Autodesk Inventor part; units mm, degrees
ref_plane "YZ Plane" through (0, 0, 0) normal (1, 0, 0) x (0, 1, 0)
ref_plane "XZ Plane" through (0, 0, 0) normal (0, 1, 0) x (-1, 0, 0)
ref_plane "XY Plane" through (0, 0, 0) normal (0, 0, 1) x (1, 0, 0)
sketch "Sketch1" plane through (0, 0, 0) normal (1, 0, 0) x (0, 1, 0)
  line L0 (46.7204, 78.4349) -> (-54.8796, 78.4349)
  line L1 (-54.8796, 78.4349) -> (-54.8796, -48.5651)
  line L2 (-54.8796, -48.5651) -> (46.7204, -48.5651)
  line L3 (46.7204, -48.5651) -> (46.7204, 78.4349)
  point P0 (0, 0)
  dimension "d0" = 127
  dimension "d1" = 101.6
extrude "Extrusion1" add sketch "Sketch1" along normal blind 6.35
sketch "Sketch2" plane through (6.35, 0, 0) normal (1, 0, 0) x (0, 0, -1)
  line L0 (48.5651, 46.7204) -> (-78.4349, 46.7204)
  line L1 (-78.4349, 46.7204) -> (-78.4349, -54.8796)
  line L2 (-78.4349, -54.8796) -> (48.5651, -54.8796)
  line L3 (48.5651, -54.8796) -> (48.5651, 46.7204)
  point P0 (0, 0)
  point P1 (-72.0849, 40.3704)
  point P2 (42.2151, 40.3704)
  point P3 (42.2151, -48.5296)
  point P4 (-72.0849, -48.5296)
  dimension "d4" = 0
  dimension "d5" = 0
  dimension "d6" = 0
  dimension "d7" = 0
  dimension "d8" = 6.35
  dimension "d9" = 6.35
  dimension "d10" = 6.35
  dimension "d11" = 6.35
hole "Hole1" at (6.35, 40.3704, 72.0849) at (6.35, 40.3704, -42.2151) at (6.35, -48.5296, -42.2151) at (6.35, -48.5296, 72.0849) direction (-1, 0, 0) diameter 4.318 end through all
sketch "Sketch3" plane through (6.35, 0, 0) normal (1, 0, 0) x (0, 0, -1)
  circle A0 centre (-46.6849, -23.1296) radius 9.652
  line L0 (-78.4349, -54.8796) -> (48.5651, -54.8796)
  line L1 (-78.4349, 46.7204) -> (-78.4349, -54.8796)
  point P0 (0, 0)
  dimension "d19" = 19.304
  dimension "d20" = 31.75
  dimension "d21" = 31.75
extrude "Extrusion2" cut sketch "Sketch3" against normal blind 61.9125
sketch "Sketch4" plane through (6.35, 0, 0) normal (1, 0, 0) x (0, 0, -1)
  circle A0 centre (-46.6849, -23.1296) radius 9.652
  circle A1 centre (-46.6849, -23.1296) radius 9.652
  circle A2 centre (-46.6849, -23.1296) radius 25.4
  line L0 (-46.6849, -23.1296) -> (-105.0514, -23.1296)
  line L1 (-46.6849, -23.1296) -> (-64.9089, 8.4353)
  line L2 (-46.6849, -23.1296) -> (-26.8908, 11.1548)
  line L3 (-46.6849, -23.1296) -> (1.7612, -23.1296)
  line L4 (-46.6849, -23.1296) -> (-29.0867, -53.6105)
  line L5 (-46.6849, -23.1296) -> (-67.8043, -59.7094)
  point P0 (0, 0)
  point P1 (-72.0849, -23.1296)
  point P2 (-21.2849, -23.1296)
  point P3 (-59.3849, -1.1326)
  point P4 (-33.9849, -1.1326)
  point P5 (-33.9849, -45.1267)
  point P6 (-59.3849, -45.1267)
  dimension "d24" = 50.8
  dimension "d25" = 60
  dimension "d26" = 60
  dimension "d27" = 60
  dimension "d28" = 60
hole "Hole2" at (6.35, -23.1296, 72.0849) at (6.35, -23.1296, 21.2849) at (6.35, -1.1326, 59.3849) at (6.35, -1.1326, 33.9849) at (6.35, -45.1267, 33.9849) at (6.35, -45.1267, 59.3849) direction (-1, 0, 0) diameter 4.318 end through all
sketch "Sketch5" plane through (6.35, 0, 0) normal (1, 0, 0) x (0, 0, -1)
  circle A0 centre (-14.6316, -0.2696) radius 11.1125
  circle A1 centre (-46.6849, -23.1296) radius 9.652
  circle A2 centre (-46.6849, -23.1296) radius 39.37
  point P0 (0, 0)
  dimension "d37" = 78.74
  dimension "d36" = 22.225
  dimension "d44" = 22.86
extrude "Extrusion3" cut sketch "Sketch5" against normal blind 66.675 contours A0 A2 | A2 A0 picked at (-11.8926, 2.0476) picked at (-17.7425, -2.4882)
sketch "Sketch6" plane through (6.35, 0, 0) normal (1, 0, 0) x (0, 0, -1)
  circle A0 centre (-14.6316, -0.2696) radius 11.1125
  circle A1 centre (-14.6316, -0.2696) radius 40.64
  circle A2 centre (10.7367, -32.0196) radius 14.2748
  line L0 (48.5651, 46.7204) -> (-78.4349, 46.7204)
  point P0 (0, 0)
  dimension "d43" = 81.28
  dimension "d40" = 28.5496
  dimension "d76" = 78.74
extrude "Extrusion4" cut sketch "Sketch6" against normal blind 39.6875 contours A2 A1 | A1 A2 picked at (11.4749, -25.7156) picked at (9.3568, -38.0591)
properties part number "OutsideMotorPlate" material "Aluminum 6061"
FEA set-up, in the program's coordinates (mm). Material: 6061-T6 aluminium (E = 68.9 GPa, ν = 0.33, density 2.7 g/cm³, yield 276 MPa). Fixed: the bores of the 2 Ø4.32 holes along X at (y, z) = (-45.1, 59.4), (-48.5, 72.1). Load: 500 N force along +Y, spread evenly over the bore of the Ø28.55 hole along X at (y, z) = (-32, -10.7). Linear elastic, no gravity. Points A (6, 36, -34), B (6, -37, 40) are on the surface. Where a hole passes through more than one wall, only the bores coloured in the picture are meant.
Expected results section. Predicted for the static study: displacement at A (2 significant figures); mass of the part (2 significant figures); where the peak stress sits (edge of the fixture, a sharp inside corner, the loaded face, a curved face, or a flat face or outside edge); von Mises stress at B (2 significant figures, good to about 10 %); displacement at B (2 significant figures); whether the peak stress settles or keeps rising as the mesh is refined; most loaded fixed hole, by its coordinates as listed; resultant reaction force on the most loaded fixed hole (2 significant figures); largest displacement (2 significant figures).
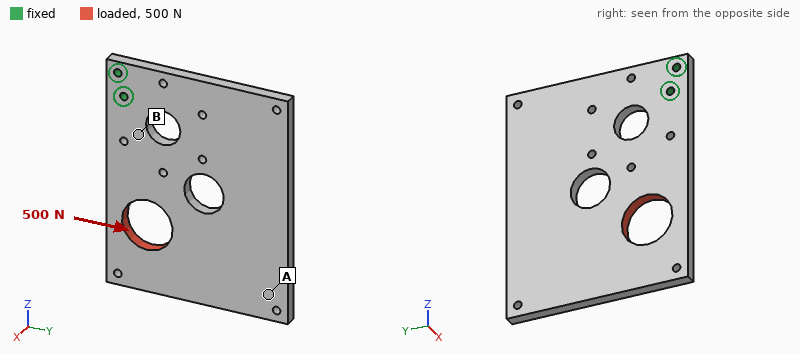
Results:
0.13 mm
200 g
edge of the fixture
11 MPa
0.024 mm
keeps rising
(-45.1, 59.4)
2.5 kN
0.15 mm
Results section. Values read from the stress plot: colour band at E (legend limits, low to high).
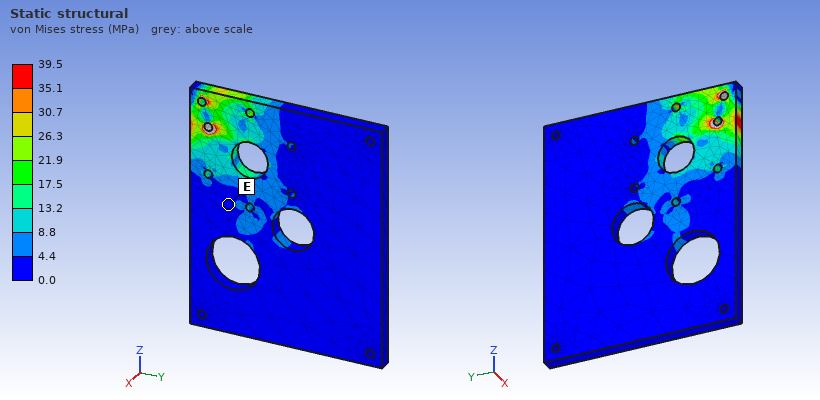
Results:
0.0 to 4.4 MPa
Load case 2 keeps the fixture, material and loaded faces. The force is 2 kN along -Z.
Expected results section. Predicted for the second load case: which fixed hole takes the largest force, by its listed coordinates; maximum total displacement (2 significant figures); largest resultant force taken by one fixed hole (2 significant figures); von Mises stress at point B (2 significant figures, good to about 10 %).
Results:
(-45.1, 59.4)
96 µm
2.4 kN
14 MPa
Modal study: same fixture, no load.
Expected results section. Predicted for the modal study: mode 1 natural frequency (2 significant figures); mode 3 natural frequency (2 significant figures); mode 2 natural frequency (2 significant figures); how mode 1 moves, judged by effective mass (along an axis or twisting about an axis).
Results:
240 Hz
850 Hz
490 Hz
along X
